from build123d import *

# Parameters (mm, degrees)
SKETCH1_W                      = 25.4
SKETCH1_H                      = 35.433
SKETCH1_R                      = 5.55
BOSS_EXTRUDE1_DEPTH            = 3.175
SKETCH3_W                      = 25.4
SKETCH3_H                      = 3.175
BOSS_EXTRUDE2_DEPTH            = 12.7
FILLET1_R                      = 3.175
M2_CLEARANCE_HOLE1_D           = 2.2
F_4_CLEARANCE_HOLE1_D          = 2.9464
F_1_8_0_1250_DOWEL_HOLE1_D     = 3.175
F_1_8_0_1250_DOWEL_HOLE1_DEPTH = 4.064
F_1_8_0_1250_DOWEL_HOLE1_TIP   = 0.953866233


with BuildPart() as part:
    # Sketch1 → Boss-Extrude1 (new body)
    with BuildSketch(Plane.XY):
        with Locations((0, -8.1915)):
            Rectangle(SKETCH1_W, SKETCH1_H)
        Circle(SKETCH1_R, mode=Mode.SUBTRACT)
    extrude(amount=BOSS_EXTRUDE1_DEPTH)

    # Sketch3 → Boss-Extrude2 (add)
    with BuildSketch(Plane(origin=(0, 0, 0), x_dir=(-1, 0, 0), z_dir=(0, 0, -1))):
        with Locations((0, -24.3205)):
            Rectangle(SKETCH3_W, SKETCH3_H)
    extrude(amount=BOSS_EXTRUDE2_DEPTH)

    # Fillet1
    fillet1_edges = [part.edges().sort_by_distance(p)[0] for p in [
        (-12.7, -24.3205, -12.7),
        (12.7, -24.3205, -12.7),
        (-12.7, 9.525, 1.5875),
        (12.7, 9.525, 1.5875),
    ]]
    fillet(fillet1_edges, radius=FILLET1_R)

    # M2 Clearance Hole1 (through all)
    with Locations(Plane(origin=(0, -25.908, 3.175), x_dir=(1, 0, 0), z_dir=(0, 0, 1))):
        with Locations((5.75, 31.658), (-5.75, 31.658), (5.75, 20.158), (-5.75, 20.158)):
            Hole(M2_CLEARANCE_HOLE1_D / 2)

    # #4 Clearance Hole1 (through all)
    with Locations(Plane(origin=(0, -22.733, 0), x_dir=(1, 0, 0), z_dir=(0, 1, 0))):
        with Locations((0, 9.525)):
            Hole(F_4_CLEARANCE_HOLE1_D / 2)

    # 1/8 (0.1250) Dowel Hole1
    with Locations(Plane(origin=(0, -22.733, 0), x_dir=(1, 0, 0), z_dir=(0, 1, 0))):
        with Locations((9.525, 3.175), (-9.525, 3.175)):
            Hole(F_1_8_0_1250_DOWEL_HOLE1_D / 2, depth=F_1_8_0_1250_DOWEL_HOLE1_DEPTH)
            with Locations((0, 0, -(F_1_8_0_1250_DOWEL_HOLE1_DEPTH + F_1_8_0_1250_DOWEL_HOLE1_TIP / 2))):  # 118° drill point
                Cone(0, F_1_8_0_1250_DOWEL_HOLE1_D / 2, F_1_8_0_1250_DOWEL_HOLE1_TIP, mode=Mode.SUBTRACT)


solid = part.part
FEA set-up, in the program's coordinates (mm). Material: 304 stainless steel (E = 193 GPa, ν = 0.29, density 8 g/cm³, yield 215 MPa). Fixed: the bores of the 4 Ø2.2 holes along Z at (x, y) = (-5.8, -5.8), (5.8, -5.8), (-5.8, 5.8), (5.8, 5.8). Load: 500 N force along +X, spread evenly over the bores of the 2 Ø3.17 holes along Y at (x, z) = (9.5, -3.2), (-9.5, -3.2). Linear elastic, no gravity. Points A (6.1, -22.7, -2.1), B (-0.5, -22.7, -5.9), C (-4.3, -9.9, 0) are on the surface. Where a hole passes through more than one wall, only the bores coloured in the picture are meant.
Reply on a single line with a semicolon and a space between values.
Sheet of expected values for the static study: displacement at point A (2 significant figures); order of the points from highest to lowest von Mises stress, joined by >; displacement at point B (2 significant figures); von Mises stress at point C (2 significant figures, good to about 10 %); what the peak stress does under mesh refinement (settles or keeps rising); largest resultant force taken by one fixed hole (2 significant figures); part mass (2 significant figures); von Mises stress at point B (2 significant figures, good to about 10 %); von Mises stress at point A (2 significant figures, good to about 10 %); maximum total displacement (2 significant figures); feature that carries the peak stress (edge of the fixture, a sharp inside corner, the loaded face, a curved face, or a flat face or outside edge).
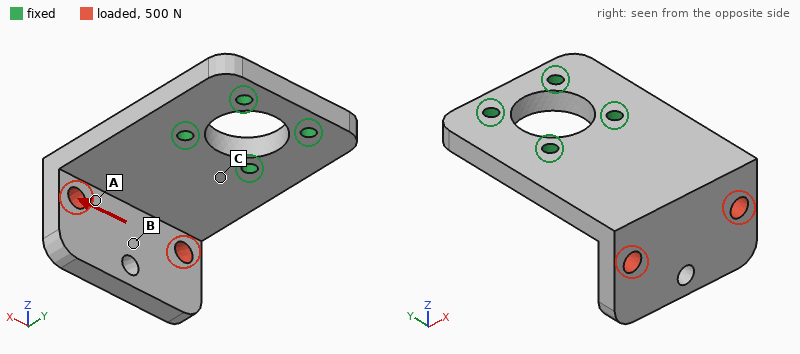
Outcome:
13 µm; C > A > B; 15 µm; 48 MPa; keeps rising; 580 N; 27 g; 12 MPa; 29 MPa; 29 µm; edge of the fixture
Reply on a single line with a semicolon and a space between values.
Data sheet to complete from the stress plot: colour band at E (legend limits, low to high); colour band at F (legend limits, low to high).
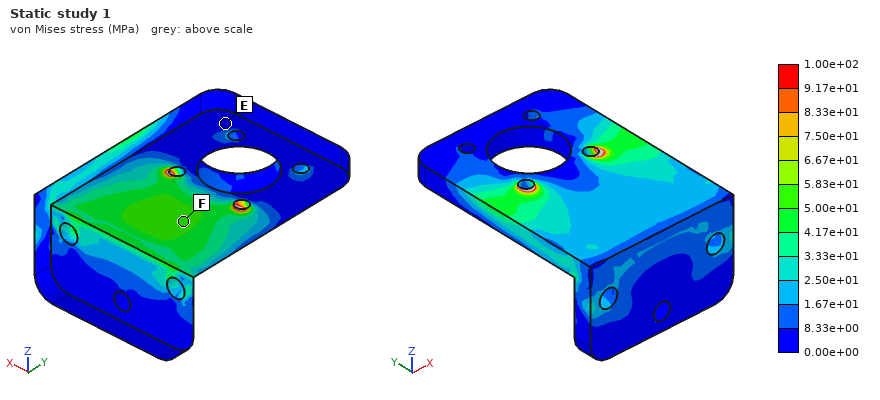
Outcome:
0.00e+00 to 8.33e+00 MPa; 5.00e+01 to 5.83e+01 MPa
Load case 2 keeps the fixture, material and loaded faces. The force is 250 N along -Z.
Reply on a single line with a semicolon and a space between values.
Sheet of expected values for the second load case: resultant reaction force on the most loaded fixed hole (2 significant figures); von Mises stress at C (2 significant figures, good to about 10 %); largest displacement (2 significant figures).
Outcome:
170 N; 82 MPa; 70 µm
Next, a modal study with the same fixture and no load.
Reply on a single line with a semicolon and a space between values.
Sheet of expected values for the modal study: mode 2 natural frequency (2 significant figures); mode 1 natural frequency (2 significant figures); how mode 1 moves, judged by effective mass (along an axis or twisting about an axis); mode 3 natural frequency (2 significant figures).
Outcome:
5700 Hz; 3000 Hz; along Z; 9400 Hz
